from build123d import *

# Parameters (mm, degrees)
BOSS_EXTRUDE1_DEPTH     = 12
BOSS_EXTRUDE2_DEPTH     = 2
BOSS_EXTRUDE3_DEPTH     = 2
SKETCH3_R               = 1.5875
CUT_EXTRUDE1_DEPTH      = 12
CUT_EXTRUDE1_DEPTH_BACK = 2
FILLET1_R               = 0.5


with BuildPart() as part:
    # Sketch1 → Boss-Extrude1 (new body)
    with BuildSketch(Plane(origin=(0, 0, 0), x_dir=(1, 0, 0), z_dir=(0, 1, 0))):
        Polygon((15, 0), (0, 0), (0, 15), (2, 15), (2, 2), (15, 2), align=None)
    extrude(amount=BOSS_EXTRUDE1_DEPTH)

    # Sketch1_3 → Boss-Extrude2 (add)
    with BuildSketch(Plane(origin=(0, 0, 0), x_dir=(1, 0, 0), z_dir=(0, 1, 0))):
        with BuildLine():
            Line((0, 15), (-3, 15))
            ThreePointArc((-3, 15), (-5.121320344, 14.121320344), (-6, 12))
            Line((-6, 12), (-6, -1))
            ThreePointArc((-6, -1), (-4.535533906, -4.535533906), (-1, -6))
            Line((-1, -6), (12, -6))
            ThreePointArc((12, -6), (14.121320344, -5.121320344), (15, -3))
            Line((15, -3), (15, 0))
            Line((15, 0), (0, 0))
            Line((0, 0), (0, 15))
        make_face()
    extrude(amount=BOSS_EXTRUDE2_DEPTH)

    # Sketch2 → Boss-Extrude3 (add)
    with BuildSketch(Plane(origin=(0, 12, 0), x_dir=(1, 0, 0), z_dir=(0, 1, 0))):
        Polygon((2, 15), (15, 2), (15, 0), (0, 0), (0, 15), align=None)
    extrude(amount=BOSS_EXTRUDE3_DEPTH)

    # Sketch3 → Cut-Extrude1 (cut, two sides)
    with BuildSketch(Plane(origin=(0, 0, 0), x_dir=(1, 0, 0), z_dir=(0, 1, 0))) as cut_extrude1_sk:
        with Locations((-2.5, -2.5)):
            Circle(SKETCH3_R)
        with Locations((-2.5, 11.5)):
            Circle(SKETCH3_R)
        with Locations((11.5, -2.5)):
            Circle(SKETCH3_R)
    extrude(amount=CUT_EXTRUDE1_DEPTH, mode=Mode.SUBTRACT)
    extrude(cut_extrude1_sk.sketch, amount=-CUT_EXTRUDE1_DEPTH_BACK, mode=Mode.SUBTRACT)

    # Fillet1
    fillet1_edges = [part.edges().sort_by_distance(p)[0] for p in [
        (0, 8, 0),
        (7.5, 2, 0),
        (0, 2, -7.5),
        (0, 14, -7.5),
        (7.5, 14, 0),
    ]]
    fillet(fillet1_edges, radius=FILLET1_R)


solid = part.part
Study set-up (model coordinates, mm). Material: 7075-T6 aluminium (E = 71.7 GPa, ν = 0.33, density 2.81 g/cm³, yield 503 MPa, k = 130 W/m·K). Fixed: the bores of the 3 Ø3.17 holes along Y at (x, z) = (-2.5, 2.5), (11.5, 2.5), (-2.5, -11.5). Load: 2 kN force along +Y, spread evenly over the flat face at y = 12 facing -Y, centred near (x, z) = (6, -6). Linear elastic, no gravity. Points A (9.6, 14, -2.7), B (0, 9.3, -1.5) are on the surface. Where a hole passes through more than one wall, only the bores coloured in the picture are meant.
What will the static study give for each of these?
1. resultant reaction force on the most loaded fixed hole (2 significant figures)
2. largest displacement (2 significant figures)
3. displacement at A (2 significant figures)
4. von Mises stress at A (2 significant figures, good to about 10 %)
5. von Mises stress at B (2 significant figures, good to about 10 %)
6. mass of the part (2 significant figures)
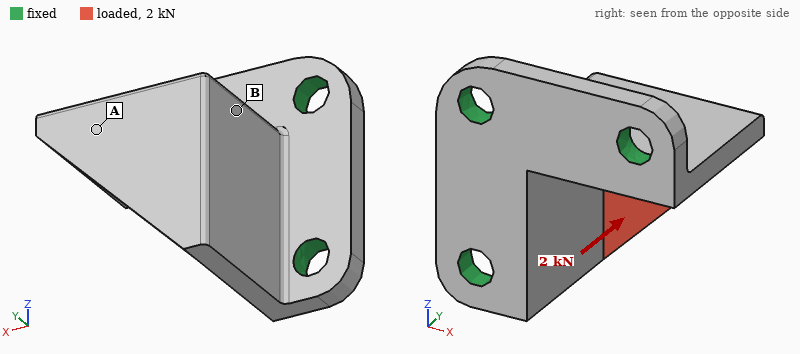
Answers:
1.1 kN
0.15 mm
0.070 mm
160 MPa
58 MPa
3.7 g
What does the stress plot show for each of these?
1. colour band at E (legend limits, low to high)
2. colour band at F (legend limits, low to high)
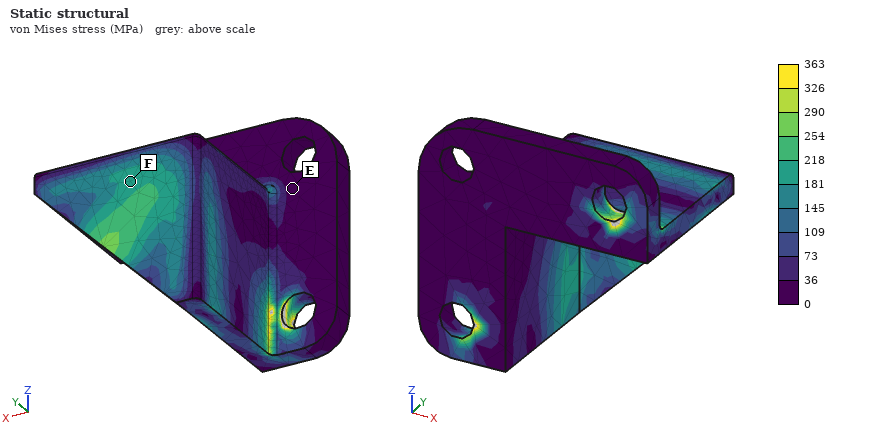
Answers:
0 to 36 MPa
181 to 218 MPa
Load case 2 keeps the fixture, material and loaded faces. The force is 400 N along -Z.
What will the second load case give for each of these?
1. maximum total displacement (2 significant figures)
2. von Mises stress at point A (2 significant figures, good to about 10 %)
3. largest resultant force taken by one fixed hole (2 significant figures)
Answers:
78 µm
55 MPa
330 N
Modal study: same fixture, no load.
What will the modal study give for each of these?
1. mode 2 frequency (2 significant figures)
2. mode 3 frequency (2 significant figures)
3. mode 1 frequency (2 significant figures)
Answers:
15 kHz
27 kHz
12 kHz
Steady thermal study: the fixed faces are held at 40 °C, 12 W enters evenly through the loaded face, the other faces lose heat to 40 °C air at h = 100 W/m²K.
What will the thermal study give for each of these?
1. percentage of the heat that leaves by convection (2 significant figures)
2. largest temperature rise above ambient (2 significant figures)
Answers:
12 %
30 K
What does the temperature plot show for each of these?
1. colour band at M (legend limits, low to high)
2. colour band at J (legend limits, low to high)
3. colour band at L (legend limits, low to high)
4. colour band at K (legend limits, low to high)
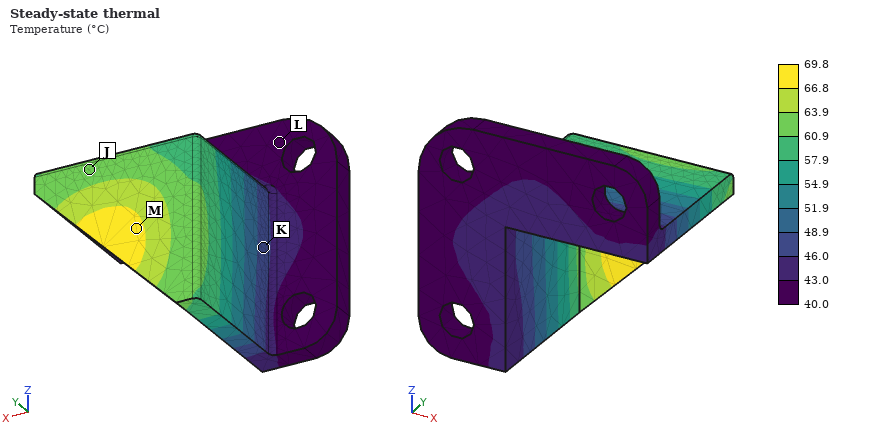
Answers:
66.8 to 69.8 °C
60.9 to 63.9 °C
40.0 to 43.0 °C
46.0 to 48.9 °C
